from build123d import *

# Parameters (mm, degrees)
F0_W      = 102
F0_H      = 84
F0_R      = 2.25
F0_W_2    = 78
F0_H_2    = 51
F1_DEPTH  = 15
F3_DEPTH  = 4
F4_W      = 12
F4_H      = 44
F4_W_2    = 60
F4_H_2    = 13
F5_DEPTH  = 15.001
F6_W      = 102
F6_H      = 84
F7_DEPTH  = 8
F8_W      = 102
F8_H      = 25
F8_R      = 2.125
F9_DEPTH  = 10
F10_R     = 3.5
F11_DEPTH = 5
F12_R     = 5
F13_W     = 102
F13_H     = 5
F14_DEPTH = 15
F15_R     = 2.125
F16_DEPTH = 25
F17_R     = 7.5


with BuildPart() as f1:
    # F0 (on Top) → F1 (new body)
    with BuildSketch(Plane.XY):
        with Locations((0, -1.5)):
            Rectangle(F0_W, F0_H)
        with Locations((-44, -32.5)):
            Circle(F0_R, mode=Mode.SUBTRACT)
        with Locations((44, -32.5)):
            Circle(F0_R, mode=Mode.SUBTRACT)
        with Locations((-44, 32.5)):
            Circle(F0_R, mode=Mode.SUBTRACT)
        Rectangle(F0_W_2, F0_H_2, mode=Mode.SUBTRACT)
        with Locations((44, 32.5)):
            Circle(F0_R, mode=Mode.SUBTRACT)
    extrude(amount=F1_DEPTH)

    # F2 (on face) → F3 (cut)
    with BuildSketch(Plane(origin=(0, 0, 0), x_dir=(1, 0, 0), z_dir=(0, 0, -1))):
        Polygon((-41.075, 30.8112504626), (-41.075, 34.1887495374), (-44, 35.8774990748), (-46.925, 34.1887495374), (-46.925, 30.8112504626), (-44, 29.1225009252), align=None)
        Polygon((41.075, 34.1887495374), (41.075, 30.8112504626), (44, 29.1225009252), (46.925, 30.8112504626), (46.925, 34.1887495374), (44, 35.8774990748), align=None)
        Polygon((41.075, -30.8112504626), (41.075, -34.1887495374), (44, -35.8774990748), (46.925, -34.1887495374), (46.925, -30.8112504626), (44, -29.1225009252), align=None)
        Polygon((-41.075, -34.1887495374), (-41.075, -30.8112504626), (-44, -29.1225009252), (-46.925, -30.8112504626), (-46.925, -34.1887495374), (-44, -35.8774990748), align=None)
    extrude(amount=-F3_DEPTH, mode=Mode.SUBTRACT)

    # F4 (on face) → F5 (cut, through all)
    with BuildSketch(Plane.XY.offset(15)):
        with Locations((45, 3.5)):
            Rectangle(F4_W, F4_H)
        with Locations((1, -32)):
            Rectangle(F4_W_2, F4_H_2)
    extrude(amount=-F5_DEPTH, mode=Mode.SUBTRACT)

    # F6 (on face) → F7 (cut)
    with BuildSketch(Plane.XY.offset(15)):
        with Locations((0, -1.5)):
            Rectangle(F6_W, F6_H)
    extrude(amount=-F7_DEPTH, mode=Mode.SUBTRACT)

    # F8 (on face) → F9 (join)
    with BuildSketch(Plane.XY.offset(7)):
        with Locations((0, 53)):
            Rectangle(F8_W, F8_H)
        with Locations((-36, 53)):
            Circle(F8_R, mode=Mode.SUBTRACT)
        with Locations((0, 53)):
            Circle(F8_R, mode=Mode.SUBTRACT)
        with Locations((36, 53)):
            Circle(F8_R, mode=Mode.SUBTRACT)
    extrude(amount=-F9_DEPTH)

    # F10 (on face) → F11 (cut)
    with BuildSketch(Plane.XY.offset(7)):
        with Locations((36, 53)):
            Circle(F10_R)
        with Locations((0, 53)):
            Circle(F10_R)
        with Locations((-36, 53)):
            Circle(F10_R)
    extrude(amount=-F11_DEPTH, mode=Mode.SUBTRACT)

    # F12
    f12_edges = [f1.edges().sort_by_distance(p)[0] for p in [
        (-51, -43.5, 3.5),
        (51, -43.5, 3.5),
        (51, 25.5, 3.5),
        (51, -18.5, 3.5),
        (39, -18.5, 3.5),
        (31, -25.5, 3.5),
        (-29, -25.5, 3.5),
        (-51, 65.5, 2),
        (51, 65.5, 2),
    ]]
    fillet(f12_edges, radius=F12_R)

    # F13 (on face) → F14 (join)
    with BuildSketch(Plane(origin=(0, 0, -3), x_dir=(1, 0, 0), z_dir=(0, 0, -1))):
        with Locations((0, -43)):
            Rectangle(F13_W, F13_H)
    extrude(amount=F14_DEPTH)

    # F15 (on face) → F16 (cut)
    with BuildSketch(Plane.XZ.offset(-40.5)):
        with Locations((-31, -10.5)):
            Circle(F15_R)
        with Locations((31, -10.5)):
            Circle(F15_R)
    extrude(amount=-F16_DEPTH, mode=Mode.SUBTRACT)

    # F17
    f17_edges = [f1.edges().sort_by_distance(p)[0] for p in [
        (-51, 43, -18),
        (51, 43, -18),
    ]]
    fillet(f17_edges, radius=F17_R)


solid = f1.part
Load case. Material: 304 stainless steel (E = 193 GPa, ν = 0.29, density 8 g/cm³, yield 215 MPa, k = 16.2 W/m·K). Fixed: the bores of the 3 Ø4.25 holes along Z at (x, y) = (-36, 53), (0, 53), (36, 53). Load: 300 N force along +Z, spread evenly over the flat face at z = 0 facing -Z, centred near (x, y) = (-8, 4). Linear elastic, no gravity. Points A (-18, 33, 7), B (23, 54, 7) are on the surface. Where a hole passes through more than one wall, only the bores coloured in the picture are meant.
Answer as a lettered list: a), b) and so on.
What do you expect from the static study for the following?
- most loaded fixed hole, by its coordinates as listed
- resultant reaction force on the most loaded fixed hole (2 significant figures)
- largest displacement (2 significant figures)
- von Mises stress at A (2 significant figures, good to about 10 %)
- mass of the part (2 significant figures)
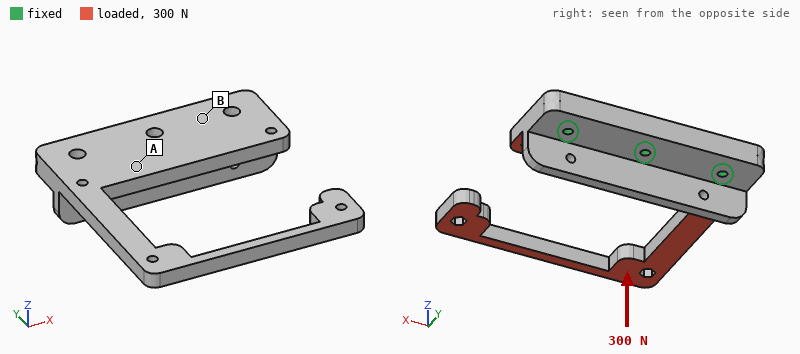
a) (0, 53)
b) 190 N
c) 1.1 mm
d) 19 MPa
e) 430 g
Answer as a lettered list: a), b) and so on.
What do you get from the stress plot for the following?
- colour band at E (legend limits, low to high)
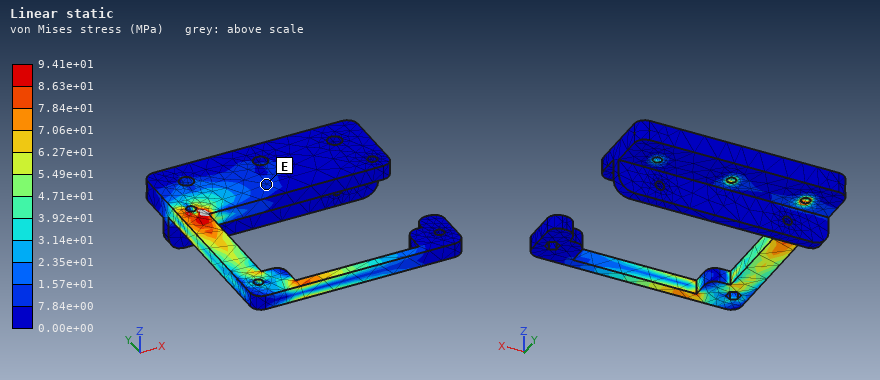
a) 7.84e+00 to 1.57e+01 MPa
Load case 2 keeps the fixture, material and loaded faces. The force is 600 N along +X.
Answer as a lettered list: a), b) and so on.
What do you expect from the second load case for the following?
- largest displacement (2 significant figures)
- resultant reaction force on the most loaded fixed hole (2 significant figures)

a) 0.25 mm
b) 580 N
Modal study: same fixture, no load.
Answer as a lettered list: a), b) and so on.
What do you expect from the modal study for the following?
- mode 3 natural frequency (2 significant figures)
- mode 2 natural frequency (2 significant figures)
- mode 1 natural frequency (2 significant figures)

a) 610 Hz
b) 280 Hz
c) 240 Hz
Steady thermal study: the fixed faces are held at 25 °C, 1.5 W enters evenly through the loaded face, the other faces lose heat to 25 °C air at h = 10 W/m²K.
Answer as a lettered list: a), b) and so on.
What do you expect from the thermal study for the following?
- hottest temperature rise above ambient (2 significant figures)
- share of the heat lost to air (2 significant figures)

a) 15 K
b) 43 %
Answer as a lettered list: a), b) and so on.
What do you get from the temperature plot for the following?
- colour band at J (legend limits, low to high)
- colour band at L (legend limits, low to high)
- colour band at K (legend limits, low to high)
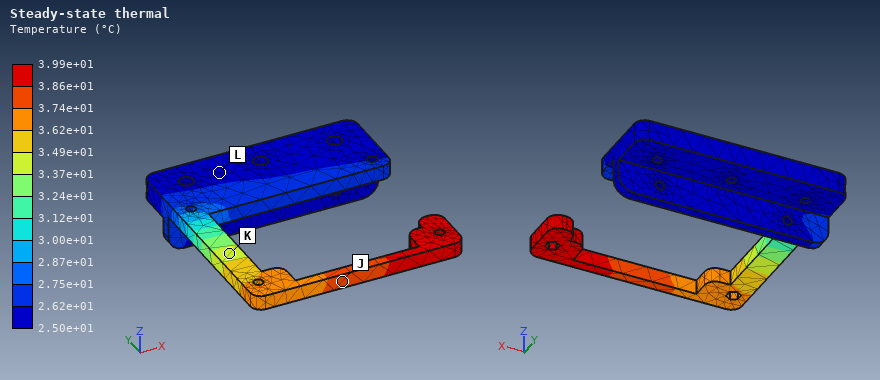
a) 3.74e+01 to 3.86e+01 °C
b) 2.50e+01 to 2.62e+01 °C
c) 3.37e+01 to 3.49e+01 °C
